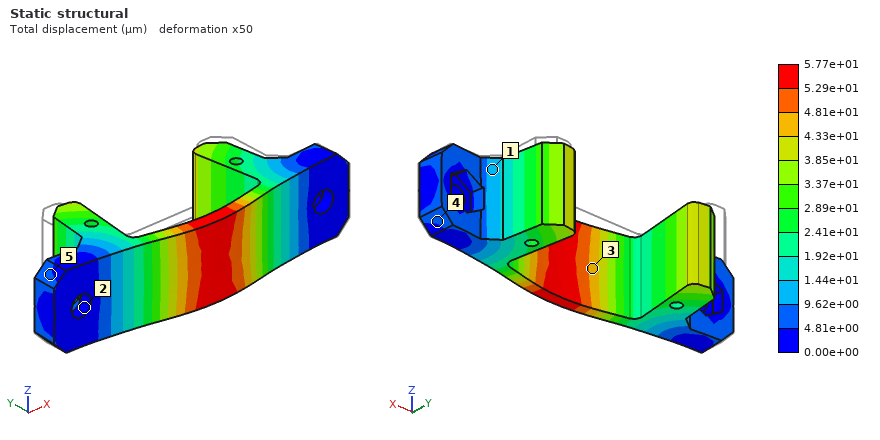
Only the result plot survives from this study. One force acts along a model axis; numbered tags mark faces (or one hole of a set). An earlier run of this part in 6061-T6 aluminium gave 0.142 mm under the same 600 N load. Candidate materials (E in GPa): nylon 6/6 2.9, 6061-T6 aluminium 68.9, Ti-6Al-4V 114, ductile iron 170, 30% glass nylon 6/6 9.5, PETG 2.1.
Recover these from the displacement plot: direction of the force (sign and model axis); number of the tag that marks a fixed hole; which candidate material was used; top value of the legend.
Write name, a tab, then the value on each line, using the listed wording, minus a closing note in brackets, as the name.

direction of the force	-Y
number of the tag that marks a fixed hole	2
which candidate material was used	ductile iron
top value of the legend	5.77e+01 µm
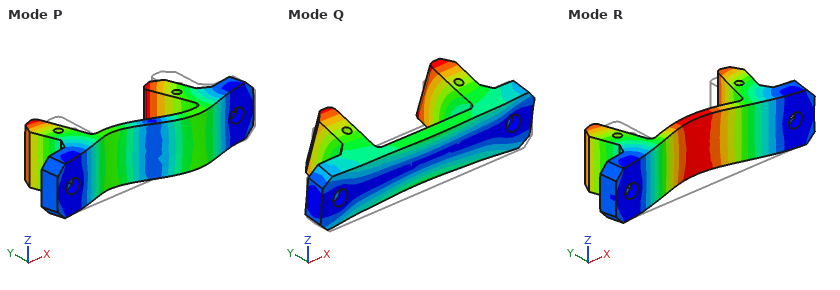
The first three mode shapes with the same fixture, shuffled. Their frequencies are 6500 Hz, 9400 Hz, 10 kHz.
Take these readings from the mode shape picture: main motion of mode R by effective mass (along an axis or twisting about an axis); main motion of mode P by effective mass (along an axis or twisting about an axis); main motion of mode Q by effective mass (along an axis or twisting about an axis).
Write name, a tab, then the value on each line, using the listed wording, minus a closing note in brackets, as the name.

main motion of mode R by effective mass	along Y
main motion of mode P by effective mass	along X
main motion of mode Q by effective mass	along Z
